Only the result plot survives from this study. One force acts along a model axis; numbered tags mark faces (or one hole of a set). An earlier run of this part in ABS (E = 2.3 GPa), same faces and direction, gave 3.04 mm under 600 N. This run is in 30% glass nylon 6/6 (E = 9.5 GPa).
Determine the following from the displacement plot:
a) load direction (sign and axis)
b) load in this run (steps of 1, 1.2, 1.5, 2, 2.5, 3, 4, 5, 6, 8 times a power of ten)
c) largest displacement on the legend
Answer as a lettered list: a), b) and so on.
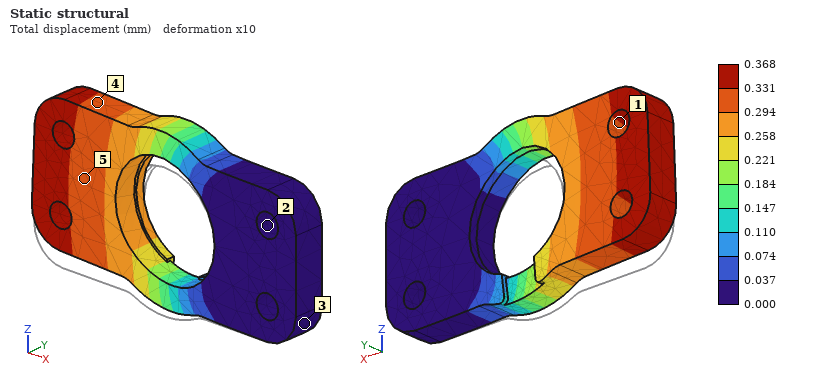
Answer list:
a) +Z
b) 300 N
c) 0.368 mm
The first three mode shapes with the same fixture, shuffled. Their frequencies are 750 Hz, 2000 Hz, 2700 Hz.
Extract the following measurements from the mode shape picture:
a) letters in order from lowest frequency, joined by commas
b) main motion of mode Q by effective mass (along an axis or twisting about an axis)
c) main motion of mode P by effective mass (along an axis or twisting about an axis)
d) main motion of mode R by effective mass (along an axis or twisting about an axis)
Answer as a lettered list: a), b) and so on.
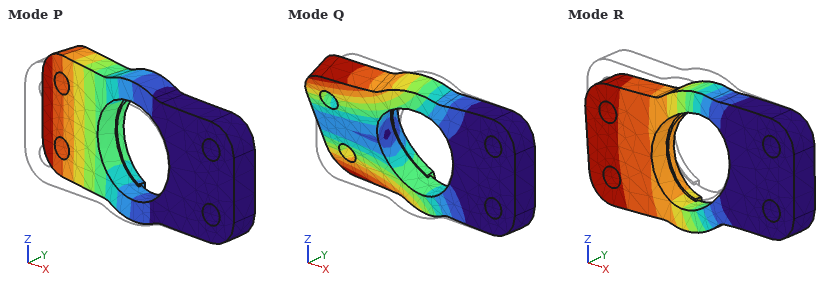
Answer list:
a) P, R, Q
b) twisting about X
c) along Y
d) along Z
